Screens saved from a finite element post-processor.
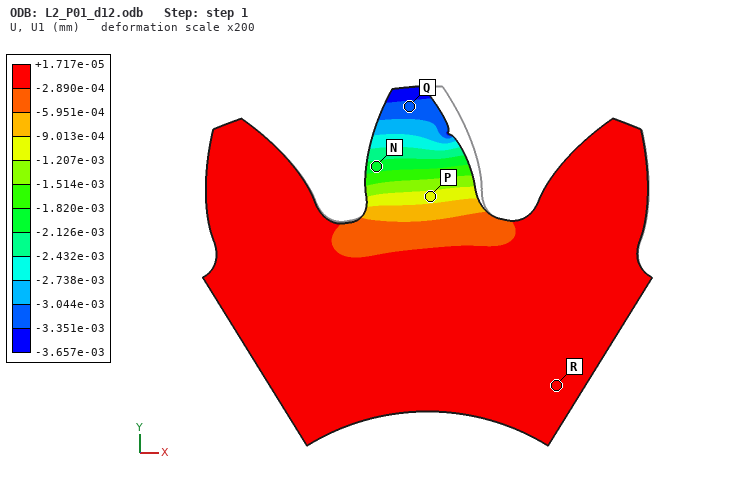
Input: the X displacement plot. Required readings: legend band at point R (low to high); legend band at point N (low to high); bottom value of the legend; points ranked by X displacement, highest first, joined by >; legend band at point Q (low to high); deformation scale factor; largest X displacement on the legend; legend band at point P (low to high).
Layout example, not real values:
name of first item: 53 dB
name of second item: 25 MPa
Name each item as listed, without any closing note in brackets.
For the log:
legend band at point R: -2.890e-04 to +1.717e-05 mm
legend band at point N: -2.126e-03 to -1.820e-03 mm
bottom value of the legend: -3.657e-03 mm
points ranked by X displacement, highest first, joined by >: R > P > N > Q
legend band at point Q: -3.351e-03 to -3.044e-03 mm
deformation scale factor: 200
largest X displacement on the legend: +1.717e-05 mm
legend band at point P: -1.207e-03 to -9.013e-04 mm
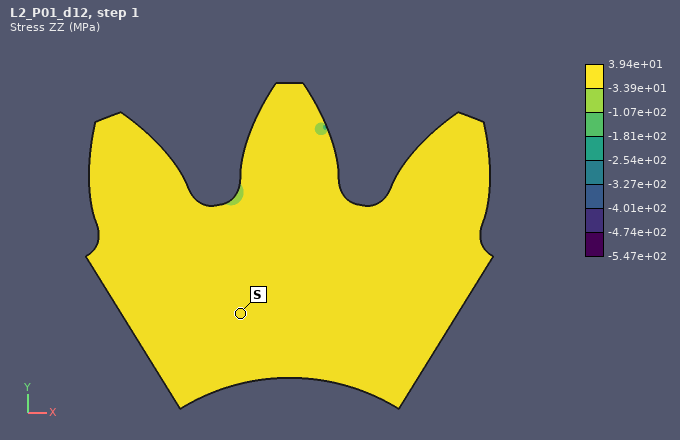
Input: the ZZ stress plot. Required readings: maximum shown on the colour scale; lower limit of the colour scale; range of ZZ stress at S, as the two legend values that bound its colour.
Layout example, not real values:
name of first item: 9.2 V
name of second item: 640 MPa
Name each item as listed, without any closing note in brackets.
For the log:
maximum shown on the colour scale: 3.94e+01 MPa
lower limit of the colour scale: -5.47e+02 MPa
range of ZZ stress at S, as the two legend values that bound its colour: -3.39e+01 to 3.94e+01 MPa
